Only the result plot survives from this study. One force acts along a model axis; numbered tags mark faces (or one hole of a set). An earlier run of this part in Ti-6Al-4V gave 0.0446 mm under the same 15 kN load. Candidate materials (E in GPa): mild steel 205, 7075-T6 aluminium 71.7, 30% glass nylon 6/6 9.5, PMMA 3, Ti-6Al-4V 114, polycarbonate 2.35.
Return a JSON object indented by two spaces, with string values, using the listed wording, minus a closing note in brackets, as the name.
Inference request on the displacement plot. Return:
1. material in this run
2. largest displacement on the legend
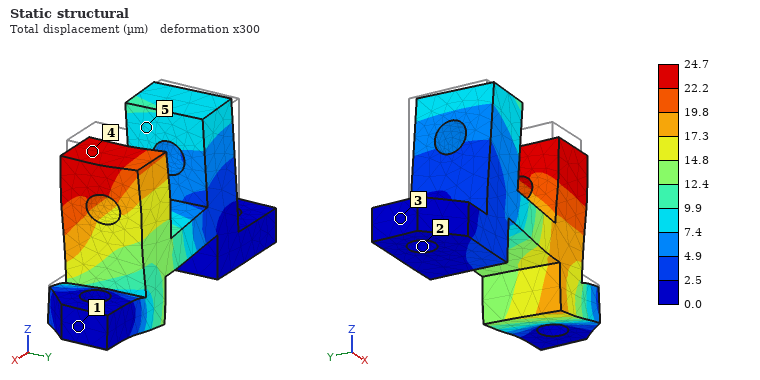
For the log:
{
  "material in this run": "mild steel",
  "largest displacement on the legend": "24.7 µm"
}
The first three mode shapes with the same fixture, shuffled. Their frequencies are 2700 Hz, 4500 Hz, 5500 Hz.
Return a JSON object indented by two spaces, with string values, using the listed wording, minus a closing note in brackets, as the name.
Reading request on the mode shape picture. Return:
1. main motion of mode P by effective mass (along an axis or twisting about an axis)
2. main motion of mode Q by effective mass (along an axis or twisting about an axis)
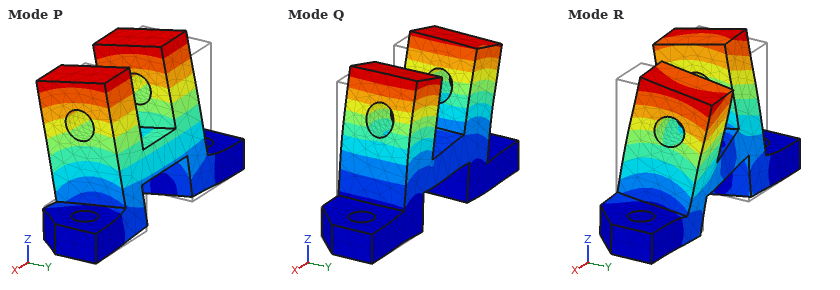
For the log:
{
  "main motion of mode P by effective mass": "along Y",
  "main motion of mode Q by effective mass": "along X"
}
